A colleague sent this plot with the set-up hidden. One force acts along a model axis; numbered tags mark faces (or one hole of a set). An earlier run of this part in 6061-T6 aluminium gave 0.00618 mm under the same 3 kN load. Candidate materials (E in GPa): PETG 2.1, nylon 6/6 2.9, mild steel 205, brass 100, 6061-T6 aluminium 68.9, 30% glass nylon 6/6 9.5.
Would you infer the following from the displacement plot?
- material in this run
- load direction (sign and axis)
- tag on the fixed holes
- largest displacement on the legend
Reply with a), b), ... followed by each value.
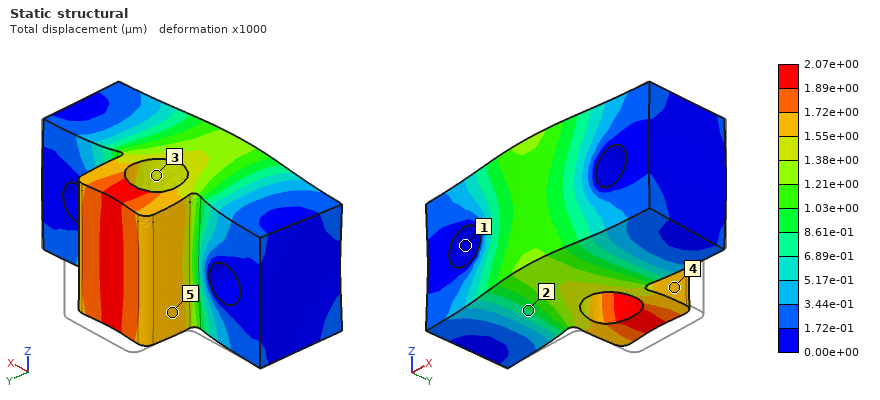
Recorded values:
a) mild steel
b) -Y
c) 1
d) 2.07e+00 µm
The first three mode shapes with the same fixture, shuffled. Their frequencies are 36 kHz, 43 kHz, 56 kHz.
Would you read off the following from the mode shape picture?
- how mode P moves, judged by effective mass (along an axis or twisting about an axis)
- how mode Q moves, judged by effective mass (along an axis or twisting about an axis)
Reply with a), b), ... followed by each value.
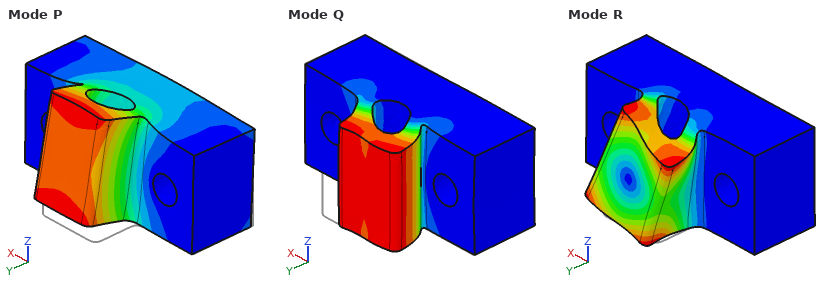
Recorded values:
a) along Z
b) along X
